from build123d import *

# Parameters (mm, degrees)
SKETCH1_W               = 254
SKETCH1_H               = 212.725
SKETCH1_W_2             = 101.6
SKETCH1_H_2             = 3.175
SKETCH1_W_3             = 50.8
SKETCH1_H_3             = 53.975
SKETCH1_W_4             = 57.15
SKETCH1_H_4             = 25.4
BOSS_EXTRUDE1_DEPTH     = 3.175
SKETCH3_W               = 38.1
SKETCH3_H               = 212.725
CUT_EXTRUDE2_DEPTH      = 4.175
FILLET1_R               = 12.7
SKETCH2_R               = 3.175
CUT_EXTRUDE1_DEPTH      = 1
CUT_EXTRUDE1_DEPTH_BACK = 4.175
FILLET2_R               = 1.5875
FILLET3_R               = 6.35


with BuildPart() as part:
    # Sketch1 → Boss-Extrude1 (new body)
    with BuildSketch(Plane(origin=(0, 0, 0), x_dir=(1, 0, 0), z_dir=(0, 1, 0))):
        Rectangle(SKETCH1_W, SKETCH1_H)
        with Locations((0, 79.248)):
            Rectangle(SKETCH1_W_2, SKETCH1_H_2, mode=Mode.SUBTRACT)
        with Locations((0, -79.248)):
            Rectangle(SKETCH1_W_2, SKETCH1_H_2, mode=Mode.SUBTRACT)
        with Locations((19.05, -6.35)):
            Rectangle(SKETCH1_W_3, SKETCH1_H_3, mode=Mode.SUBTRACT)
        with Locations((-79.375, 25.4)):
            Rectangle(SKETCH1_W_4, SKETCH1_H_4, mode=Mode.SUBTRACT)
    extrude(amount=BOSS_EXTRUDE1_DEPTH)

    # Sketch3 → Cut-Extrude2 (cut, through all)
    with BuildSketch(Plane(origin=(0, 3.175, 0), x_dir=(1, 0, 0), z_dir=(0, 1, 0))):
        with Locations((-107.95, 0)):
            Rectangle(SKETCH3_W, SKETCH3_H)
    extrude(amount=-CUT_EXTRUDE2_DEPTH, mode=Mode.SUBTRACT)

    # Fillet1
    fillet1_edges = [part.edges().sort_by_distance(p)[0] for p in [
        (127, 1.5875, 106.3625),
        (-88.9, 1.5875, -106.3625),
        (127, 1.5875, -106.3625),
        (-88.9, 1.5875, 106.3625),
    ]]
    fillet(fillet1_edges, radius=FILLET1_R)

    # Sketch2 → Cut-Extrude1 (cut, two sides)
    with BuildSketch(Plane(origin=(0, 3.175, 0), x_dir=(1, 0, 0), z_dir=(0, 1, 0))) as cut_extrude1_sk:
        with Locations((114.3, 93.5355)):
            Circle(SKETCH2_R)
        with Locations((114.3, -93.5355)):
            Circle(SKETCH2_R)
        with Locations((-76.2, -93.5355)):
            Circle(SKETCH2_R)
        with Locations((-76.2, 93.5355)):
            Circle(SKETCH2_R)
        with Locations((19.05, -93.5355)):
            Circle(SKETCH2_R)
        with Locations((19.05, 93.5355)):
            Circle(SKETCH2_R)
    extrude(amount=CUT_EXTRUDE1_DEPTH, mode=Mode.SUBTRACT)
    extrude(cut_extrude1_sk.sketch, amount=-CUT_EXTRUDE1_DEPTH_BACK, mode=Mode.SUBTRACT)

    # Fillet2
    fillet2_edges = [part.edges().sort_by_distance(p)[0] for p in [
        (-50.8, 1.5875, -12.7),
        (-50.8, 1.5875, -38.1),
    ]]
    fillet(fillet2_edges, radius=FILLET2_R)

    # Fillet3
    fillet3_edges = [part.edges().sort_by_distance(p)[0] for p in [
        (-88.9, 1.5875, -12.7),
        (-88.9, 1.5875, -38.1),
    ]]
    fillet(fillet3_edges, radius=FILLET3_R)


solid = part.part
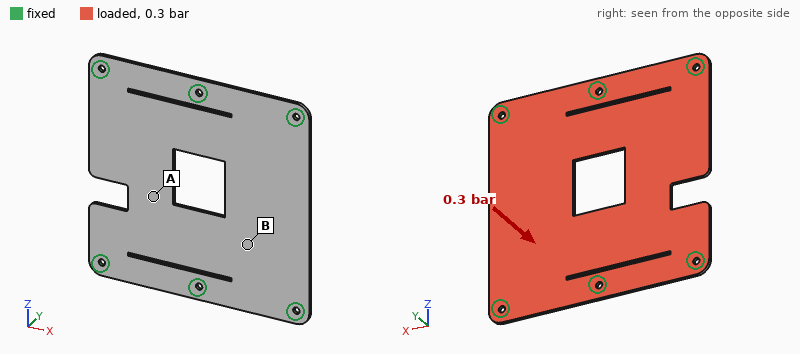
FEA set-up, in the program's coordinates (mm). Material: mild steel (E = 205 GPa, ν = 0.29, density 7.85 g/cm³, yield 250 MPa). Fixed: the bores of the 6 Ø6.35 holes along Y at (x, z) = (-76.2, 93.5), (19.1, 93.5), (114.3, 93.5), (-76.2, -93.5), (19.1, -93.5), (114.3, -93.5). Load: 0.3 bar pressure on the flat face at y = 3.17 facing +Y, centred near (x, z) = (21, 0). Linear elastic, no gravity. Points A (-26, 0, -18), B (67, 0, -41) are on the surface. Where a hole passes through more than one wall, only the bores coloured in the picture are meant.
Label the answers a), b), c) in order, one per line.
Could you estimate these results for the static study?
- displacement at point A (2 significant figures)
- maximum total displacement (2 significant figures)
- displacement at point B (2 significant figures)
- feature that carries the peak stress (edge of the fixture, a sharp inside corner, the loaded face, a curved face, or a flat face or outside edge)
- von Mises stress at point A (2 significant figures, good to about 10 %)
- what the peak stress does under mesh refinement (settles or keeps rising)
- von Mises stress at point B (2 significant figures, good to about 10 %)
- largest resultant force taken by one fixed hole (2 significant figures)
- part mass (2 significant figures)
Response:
a) 0.37 mm
b) 0.43 mm
c) 0.25 mm
d) edge of the fixture
e) 41 MPa
f) keeps rising
g) 20 MPa
h) 220 N
i) 1.0 kg
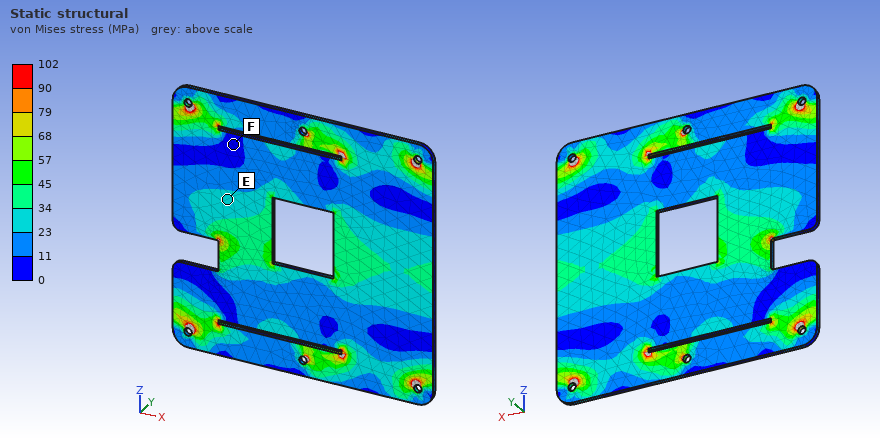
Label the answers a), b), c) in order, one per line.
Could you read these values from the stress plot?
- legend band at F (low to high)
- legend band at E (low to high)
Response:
a) 0 to 11 MPa
b) 23 to 34 MPa
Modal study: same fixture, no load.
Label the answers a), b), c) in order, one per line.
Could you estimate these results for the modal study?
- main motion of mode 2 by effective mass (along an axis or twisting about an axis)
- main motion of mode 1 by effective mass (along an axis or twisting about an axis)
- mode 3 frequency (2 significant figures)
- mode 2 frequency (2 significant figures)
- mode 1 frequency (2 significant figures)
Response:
a) twisting about Z
b) along Y
c) 690 Hz
d) 490 Hz
e) 340 Hz
